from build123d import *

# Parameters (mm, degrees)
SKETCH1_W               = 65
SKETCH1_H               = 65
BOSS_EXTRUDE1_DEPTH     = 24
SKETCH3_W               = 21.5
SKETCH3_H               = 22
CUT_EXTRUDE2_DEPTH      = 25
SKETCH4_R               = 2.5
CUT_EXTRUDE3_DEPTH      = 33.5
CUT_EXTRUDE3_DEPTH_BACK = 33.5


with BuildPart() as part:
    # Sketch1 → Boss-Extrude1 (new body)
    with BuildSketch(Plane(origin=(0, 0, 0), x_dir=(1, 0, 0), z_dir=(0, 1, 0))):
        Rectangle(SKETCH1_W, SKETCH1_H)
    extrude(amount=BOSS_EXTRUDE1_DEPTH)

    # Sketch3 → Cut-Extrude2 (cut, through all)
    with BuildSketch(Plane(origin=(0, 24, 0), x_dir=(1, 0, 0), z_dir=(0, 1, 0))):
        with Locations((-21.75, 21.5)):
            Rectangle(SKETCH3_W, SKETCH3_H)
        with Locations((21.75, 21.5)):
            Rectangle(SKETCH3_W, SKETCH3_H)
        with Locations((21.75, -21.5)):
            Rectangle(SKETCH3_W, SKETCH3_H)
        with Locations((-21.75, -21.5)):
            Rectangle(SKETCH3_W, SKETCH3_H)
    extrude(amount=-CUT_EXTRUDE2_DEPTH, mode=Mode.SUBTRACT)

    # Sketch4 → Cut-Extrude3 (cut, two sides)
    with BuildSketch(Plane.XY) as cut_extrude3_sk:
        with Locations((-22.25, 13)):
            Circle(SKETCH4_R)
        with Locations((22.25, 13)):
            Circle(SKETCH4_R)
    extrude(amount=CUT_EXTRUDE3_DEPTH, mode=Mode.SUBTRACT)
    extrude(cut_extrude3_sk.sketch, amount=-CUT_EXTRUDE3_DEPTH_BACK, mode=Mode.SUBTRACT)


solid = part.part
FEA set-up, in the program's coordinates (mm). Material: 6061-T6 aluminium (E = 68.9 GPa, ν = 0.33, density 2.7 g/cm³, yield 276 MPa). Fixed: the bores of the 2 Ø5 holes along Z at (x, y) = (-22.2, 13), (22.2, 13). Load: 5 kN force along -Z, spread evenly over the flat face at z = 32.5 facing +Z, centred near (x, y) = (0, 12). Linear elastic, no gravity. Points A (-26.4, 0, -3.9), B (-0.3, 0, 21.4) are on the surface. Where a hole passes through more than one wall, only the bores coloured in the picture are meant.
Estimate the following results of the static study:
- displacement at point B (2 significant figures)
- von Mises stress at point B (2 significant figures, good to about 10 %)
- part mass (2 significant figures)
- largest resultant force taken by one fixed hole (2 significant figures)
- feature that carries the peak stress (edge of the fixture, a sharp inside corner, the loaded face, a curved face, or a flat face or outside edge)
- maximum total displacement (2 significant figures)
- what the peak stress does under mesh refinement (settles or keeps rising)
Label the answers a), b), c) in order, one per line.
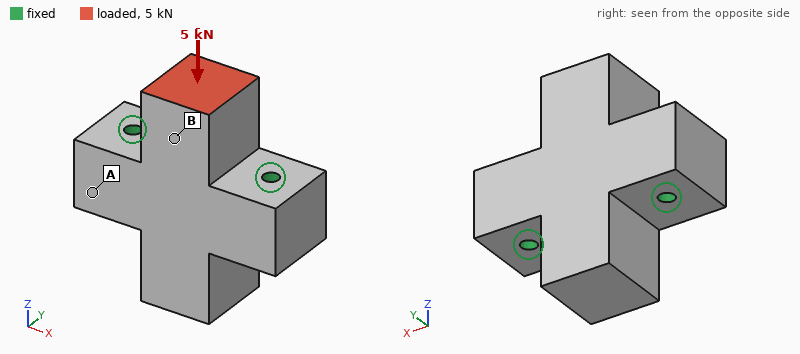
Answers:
a) 6.4 µm
b) 8.9 MPa
c) 150 g
d) 2.5 kN
e) edge of the fixture
f) 8.0 µm
g) keeps rising
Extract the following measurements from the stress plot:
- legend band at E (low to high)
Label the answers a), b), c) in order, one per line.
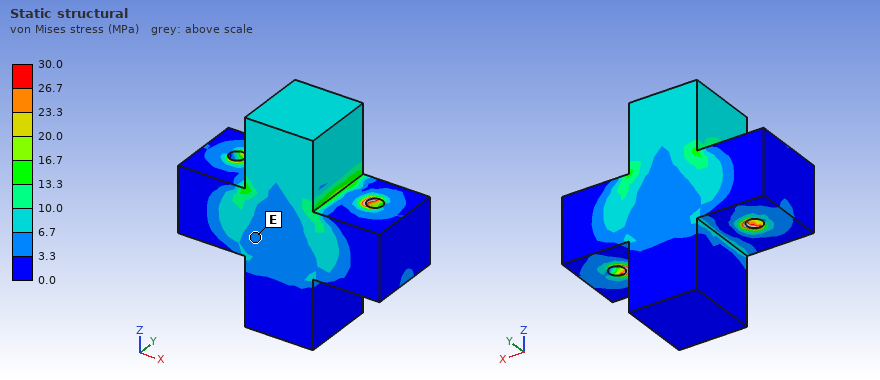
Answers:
a) 3.3 to 6.7 MPa
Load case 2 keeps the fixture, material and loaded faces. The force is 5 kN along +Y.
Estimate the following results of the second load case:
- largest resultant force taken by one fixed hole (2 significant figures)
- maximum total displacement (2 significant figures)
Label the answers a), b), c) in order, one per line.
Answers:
a) 2.5 kN
b) 91 µm
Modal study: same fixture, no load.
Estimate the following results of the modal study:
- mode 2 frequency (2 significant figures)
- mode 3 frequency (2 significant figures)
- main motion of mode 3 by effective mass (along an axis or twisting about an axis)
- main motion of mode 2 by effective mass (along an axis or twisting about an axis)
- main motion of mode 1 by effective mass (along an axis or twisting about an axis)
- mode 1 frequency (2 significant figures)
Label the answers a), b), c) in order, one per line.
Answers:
a) 11 kHz
b) 15 kHz
c) twisting about Y
d) along Y
e) twisting about X
f) 8300 Hz
